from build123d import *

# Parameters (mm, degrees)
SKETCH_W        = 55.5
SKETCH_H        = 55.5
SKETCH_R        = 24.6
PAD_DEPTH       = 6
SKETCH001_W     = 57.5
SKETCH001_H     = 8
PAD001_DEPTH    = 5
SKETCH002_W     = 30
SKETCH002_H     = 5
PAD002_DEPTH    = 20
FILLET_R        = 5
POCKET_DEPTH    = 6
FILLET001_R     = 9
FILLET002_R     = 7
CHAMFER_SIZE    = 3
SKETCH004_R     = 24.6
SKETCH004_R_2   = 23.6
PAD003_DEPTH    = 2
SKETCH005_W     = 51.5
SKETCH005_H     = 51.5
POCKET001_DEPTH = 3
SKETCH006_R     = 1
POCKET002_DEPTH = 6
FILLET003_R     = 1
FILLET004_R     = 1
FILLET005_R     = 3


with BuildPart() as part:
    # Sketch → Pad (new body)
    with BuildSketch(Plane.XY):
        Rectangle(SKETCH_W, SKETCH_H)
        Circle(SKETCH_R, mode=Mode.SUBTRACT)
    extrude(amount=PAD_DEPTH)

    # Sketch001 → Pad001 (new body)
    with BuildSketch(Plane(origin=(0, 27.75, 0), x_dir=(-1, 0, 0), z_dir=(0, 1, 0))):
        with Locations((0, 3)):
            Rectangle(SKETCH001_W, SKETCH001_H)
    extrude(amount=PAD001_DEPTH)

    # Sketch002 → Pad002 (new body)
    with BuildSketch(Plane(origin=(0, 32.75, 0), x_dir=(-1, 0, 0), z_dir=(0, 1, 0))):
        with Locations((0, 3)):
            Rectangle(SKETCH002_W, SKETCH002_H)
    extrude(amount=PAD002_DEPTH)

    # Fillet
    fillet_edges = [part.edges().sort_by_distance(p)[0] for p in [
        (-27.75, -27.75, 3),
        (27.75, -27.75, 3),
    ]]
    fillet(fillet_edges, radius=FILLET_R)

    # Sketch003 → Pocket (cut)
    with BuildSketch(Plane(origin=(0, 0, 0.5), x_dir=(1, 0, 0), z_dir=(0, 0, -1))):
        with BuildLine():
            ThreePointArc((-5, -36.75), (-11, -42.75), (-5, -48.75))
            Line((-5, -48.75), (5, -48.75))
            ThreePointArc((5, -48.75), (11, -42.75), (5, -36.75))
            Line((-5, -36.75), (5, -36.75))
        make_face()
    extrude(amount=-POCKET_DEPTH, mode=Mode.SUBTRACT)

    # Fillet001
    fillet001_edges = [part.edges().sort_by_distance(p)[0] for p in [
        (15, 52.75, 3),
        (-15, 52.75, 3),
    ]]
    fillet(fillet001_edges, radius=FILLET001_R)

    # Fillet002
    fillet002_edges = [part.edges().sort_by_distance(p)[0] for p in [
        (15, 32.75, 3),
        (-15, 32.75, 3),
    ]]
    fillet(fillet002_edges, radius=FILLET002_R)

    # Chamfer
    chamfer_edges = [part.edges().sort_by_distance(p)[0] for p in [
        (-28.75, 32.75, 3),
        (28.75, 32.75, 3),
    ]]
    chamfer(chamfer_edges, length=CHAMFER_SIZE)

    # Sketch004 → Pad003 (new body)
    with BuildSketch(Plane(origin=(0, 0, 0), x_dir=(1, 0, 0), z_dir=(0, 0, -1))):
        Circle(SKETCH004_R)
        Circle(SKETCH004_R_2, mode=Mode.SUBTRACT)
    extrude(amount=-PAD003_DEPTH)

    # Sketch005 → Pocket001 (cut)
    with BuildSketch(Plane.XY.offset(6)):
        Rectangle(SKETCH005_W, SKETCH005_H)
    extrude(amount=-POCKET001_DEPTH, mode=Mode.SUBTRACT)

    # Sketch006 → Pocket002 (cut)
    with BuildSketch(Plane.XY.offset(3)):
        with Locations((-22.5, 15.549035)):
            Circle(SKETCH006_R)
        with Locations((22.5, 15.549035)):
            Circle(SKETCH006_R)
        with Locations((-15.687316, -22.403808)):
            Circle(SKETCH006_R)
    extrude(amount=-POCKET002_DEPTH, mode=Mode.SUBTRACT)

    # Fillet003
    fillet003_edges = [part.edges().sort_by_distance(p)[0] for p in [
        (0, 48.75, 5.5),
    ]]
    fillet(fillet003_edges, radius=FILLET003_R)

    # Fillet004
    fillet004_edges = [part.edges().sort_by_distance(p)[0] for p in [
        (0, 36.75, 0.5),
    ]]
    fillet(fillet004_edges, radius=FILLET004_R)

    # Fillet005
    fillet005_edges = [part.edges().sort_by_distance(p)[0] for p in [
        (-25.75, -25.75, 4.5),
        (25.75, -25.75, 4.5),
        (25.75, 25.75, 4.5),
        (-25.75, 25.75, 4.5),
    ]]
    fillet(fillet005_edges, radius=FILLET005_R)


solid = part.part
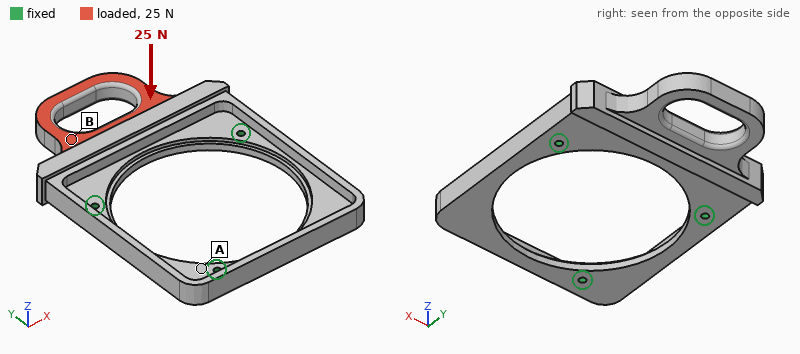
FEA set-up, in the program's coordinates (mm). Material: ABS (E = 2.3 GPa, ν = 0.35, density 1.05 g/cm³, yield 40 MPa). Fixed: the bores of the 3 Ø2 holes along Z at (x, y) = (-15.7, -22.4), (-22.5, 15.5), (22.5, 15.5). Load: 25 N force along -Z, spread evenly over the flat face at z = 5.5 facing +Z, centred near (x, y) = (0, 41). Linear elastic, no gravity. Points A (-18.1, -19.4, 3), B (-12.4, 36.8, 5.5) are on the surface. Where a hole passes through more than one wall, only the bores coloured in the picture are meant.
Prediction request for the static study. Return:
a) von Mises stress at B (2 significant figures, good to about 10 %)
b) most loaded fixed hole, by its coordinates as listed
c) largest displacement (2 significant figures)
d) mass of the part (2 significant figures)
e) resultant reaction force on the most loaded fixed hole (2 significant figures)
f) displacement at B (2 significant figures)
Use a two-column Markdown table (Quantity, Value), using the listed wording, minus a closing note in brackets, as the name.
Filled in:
| Quantity | Value |
|---|---|
| von Mises stress at B | 2.6 MPa |
| most loaded fixed hole, by its coordinates as listed | (-22.5, 15.5) |
| largest displacement | 1.0 mm |
| mass of the part | 9.5 g |
| resultant reaction force on the most loaded fixed hole | 17 N |
| displacement at B | 0.51 mm |
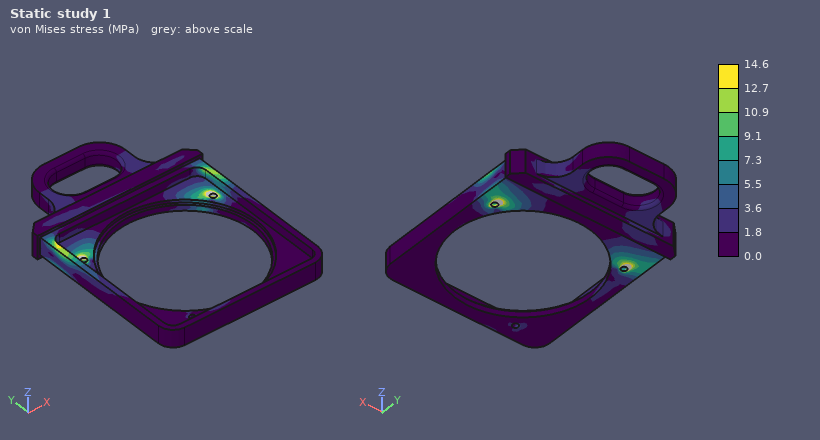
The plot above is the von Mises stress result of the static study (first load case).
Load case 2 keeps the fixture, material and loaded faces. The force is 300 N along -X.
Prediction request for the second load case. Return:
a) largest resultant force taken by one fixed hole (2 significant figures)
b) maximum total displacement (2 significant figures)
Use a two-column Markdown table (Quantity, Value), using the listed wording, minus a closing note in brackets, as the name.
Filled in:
| Quantity | Value |
|---|---|
| largest resultant force taken by one fixed hole | 220 N |
| maximum total displacement | 0.43 mm |
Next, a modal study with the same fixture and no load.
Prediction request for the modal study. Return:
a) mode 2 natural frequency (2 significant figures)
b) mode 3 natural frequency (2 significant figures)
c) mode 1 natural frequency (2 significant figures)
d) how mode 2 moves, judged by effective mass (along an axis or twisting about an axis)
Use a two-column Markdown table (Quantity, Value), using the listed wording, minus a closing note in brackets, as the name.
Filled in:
| Quantity | Value |
|---|---|
| mode 2 natural frequency | 700 Hz |
| mode 3 natural frequency | 2100 Hz |
| mode 1 natural frequency | 570 Hz |
| how mode 2 moves, judged by effective mass | along Z |
